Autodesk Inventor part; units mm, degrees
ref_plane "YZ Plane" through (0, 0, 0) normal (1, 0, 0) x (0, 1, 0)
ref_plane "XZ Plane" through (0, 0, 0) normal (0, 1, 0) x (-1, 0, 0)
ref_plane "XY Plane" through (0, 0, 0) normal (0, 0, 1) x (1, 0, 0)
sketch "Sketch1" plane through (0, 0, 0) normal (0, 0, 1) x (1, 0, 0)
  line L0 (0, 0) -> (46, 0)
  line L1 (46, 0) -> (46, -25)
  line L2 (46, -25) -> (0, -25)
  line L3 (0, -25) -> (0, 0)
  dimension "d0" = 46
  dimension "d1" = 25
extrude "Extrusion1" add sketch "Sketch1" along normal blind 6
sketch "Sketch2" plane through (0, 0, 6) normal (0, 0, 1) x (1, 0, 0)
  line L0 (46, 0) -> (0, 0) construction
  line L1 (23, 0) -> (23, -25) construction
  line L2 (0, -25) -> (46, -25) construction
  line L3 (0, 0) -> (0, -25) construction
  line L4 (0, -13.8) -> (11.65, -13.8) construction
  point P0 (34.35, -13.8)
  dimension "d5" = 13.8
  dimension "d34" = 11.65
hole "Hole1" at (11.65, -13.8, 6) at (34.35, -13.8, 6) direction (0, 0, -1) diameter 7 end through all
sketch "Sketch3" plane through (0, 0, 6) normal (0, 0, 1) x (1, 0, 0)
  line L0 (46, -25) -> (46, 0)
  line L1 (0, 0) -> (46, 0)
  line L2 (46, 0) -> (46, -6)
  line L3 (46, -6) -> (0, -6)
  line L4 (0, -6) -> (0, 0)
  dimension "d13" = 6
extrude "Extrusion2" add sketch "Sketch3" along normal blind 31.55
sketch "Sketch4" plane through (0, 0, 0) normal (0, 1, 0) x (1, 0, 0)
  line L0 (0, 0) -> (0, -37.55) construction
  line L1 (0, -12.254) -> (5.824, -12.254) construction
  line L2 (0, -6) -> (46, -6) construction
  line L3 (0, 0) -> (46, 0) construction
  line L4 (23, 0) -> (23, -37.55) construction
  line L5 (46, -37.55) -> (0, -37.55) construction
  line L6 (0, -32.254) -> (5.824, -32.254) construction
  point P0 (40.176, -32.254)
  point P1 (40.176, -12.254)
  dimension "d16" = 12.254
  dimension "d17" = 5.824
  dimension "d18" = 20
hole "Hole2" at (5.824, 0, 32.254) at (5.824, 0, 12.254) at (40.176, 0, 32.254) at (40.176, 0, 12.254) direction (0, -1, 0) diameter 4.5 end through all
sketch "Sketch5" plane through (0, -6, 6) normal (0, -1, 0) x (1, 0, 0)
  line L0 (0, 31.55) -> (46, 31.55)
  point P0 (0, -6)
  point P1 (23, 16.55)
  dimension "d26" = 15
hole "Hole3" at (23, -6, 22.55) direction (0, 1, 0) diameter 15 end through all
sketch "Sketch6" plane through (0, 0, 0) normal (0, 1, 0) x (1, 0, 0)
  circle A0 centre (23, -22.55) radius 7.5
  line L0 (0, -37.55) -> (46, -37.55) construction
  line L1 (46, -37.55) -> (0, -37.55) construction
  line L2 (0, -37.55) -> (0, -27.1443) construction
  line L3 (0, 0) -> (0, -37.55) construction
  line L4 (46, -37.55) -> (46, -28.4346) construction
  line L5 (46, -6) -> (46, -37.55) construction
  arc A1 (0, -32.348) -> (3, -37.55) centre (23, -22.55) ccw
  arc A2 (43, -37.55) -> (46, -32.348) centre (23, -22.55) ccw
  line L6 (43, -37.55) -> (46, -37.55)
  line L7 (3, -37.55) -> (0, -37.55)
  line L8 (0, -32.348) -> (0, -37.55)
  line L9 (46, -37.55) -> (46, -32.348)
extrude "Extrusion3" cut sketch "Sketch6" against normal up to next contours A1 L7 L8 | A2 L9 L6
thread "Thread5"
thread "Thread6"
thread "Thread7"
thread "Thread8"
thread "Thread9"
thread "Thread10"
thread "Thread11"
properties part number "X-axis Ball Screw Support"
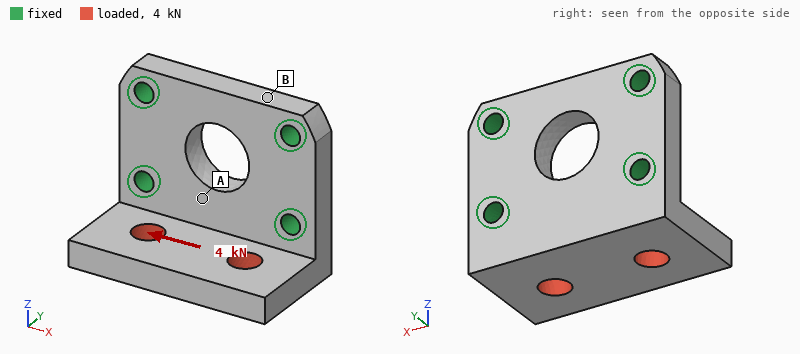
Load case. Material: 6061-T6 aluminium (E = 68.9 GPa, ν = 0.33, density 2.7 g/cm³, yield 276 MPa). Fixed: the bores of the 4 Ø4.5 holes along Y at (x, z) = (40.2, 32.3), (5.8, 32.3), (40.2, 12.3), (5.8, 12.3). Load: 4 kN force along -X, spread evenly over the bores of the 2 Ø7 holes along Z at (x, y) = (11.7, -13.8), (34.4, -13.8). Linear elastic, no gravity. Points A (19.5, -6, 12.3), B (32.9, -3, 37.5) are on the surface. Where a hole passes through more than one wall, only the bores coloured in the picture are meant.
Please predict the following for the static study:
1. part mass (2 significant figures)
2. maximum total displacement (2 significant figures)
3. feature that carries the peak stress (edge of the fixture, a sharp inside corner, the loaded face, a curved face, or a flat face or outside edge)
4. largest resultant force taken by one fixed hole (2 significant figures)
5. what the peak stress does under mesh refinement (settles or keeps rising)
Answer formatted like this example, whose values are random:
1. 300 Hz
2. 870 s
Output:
1. 37 g
2. 40 µm
3. edge of the fixture
4. 2.5 kN
5. keeps rising
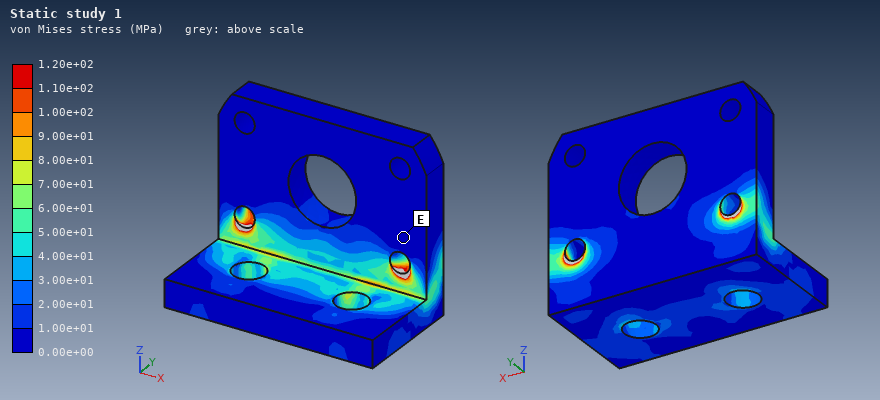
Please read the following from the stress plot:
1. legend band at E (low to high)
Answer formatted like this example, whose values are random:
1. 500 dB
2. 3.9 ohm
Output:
1. 0.00e+00 to 1.00e+01 MPa
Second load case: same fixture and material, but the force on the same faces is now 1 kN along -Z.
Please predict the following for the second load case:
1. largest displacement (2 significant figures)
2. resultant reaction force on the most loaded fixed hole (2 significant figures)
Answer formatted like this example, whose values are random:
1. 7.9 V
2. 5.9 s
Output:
1. 59 µm
2. 410 N
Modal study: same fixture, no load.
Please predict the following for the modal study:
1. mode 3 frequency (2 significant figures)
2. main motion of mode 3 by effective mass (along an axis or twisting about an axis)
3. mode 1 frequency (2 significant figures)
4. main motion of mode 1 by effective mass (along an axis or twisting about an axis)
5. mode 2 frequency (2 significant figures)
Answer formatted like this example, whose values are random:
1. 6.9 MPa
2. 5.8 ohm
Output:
1. 16 kHz
2. along X
3. 6000 Hz
4. along Z
5. 10 kHz
